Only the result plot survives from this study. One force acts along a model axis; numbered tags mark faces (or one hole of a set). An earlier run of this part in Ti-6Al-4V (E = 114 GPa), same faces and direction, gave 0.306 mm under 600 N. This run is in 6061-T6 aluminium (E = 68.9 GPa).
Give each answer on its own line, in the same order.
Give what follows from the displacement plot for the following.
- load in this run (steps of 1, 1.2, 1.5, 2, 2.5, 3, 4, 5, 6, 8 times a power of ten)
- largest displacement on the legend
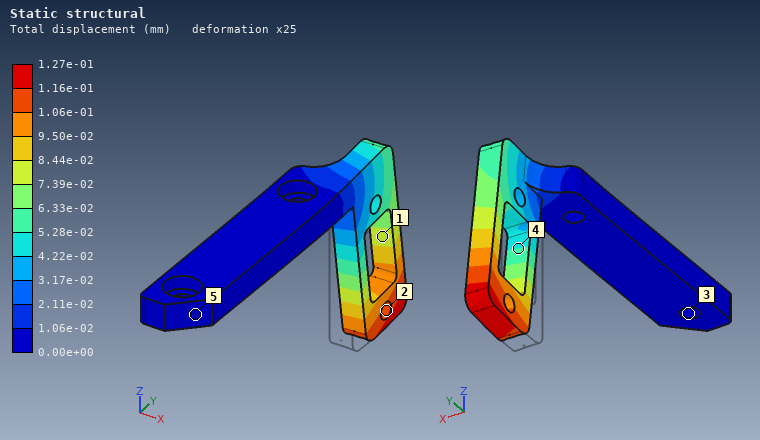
150 N
1.27e-01 mm
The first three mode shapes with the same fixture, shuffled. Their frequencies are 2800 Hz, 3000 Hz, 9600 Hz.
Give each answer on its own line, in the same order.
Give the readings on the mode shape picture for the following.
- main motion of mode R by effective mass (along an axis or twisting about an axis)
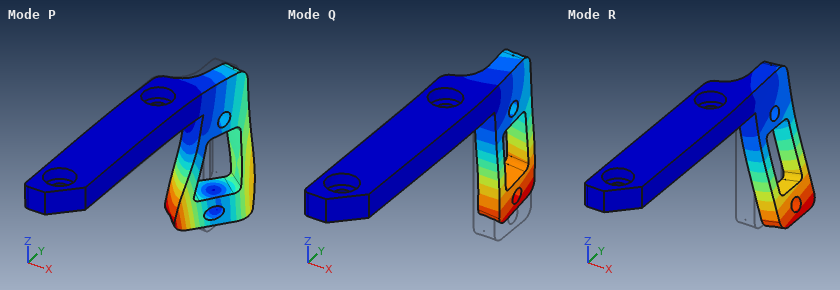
along X
